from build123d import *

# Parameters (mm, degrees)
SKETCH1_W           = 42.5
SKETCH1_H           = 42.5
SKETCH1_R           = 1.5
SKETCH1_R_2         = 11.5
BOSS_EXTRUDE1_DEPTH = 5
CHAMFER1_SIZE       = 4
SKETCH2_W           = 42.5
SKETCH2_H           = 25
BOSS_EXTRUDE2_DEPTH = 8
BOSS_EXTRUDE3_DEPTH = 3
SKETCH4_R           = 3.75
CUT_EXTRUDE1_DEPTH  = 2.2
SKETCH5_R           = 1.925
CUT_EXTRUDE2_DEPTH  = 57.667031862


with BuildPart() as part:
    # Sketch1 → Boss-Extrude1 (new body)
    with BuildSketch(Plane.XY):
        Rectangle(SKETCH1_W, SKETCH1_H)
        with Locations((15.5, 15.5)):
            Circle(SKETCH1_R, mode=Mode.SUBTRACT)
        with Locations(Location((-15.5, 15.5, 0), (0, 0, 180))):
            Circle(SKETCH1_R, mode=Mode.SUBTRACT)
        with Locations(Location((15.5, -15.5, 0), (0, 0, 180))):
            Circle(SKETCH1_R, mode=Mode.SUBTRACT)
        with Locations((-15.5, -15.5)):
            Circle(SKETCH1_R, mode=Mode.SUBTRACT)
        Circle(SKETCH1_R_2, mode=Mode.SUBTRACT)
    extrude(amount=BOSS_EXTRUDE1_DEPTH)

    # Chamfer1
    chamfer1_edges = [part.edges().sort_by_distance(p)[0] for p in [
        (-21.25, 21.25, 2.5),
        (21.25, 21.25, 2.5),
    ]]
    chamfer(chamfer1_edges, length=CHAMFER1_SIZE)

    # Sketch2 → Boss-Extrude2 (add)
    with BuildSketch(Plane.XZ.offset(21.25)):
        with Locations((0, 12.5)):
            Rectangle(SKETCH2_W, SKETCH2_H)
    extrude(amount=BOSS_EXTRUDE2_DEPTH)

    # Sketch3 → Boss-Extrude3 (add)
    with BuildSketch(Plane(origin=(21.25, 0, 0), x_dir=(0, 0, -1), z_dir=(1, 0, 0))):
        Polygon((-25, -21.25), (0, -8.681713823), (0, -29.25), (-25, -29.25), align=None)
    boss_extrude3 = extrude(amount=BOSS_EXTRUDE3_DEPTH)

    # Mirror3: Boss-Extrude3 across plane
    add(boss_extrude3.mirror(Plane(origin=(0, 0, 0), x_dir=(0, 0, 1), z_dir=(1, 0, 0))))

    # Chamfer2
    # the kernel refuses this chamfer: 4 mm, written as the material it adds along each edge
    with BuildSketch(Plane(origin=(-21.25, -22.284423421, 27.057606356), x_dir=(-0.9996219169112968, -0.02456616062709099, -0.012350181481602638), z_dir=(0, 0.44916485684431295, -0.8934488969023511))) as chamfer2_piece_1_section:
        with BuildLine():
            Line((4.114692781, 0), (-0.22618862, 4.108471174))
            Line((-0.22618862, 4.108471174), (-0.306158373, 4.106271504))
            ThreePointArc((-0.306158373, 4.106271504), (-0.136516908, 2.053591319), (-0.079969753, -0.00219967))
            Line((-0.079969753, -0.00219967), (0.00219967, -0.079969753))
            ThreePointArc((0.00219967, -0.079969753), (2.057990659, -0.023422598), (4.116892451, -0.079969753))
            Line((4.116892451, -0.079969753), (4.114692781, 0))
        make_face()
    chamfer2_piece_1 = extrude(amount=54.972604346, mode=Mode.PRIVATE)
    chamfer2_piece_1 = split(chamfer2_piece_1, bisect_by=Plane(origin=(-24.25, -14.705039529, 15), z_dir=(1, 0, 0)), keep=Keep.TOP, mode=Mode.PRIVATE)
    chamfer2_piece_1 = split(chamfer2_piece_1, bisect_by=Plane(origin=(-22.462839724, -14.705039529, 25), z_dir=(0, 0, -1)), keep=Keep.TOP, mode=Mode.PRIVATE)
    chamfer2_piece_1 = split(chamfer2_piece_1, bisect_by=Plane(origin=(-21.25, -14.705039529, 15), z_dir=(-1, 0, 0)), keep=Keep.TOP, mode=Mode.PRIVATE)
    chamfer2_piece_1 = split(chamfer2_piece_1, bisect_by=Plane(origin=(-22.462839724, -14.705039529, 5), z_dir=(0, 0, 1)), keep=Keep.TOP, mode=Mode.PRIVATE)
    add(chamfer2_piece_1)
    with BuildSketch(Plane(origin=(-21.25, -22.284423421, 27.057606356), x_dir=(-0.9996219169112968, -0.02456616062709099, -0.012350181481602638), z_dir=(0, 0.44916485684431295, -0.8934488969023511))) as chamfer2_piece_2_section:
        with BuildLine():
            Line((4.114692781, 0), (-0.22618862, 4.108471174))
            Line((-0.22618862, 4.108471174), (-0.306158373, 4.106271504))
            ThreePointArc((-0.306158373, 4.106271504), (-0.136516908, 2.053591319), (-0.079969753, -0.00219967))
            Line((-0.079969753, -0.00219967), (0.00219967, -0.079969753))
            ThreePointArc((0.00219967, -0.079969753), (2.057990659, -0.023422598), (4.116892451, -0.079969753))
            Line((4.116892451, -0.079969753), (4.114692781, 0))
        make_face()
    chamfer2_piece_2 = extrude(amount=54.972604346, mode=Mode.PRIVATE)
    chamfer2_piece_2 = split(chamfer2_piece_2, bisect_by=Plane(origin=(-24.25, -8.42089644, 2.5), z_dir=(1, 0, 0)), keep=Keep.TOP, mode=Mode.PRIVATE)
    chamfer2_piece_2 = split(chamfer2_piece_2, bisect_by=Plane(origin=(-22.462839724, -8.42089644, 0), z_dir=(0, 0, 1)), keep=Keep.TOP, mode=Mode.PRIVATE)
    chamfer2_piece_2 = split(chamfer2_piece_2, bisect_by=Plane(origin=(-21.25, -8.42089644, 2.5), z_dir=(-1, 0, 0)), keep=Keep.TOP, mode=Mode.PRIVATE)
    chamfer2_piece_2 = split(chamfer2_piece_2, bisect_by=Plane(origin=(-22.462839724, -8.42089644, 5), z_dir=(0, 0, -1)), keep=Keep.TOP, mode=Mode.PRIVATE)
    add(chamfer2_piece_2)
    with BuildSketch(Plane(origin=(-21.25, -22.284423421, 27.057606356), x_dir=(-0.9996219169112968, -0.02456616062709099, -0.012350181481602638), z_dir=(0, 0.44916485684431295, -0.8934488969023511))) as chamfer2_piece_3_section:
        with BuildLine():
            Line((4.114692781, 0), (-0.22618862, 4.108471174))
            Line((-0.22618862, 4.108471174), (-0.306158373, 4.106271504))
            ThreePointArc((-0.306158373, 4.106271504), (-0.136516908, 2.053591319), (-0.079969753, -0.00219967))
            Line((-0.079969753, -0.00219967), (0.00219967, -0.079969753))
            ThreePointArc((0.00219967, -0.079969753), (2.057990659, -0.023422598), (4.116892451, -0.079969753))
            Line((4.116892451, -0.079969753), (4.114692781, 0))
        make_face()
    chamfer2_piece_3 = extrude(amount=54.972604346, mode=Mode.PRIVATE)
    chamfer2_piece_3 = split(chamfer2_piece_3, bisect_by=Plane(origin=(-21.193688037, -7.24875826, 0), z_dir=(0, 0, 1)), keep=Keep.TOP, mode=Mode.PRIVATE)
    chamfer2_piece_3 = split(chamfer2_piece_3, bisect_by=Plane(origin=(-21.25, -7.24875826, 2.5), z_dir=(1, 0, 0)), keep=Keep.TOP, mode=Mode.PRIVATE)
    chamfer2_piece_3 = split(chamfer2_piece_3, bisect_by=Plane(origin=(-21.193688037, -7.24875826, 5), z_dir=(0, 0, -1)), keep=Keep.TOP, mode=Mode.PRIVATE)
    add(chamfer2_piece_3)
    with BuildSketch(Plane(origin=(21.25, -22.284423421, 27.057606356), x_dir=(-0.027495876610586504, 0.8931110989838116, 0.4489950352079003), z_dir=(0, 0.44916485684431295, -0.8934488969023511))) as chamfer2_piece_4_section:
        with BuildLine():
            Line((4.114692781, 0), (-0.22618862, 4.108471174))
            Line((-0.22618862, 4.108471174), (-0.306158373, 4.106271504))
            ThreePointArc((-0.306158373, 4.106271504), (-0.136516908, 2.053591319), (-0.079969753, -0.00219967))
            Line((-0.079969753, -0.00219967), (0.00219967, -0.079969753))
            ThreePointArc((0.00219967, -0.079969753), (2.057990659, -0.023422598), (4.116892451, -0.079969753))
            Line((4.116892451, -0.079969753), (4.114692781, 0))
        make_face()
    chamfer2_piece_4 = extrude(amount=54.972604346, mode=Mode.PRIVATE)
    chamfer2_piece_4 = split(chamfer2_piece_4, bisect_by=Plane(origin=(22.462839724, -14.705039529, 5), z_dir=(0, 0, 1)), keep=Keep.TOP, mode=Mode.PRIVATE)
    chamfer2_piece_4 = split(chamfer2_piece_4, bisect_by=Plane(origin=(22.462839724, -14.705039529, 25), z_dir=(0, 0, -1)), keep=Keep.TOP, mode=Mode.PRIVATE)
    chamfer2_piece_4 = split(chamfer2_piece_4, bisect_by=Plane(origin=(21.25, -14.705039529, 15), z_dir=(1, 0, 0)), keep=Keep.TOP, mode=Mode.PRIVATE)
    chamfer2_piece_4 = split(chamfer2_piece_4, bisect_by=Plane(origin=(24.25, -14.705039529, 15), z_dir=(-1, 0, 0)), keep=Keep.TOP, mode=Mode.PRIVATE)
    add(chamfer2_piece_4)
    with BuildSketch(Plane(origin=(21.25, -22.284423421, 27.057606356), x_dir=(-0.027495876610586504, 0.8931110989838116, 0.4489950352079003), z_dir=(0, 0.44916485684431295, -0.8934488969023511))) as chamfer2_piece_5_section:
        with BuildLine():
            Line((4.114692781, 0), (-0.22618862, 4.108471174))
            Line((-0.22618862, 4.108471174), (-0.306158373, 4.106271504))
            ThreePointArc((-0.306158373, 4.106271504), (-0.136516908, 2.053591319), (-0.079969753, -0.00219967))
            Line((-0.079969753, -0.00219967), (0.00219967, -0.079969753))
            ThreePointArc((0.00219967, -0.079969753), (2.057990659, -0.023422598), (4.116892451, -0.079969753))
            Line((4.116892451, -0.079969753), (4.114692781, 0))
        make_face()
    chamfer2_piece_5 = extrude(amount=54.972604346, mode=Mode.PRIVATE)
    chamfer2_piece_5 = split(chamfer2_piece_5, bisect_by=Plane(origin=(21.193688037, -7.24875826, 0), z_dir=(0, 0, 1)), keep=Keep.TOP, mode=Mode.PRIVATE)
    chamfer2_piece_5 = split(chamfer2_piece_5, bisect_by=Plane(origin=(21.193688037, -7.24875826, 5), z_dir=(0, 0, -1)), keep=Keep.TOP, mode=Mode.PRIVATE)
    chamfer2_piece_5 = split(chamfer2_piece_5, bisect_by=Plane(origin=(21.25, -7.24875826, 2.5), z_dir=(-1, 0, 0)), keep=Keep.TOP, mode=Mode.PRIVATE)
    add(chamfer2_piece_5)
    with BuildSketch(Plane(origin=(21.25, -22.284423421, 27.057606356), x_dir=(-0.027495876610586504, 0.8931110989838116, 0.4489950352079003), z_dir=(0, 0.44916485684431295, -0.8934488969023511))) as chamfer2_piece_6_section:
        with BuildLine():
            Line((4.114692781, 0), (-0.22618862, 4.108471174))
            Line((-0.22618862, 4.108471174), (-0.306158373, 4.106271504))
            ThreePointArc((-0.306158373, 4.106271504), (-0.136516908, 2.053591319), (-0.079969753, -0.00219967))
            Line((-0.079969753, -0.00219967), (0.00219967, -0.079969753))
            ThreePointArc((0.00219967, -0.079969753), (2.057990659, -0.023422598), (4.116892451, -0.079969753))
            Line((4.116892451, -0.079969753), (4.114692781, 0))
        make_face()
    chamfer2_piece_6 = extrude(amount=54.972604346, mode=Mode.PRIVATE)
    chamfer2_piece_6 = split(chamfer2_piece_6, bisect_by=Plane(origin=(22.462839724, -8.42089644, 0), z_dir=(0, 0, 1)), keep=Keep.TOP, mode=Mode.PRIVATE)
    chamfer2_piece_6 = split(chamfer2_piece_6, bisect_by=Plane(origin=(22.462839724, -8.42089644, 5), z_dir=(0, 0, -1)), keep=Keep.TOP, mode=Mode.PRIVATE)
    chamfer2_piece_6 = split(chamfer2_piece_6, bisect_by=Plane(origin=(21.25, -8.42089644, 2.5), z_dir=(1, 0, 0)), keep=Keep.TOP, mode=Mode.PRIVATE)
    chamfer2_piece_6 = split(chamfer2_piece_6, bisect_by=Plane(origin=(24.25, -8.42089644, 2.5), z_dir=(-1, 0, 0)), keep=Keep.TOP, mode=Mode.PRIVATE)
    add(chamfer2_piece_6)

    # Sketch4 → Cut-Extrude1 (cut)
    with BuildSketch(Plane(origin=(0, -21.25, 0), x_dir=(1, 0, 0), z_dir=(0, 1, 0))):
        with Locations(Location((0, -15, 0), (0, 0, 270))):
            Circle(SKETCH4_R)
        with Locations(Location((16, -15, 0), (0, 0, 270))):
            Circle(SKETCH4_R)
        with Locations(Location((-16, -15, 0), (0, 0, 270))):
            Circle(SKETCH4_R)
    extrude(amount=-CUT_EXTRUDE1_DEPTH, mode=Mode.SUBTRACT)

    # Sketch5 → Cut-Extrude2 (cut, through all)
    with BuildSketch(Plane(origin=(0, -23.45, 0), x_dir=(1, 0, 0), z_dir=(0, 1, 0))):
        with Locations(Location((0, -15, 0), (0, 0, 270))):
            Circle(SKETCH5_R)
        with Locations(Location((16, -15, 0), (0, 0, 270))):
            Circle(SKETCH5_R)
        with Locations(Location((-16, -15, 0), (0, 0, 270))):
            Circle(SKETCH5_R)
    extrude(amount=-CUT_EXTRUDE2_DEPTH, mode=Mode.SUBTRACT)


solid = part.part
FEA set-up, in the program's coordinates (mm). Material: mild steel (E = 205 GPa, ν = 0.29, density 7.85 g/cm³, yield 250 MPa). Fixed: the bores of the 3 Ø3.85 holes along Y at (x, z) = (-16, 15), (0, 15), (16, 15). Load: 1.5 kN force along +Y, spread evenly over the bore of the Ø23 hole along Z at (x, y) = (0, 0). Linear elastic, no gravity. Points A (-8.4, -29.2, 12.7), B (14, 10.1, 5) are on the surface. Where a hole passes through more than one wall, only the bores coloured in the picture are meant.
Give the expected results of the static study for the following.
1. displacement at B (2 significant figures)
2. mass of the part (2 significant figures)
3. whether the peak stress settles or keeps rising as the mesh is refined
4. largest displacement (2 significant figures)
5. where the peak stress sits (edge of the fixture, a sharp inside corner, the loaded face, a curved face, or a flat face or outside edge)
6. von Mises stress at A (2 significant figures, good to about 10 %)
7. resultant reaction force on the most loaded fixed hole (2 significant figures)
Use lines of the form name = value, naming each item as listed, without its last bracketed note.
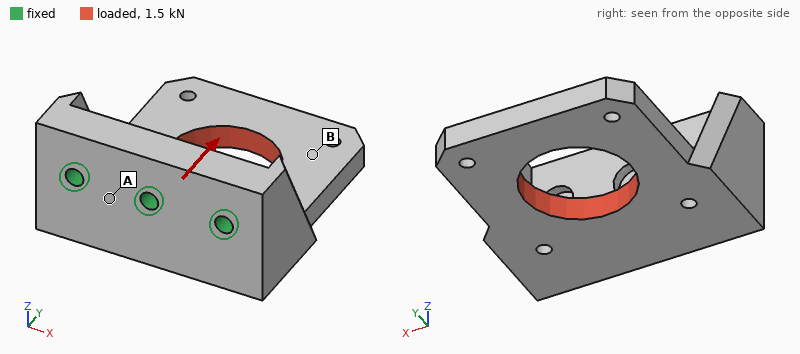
displacement at B = 15 µm
mass of the part = 140 g
whether the peak stress settles or keeps rising as the mesh is refined = keeps rising
largest displacement = 21 µm
where the peak stress sits = edge of the fixture
von Mises stress at A = 16 MPa
resultant reaction force on the most loaded fixed hole = 540 N
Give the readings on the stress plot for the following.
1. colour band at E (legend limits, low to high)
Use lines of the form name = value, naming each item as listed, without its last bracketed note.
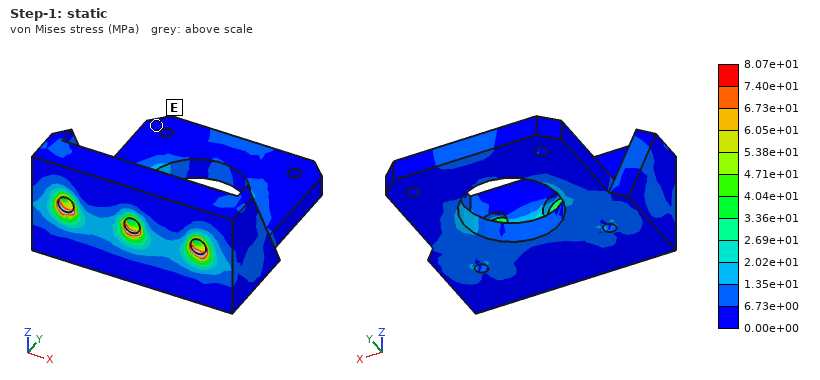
colour band at E = 0.00e+00 to 6.73e+00 MPa
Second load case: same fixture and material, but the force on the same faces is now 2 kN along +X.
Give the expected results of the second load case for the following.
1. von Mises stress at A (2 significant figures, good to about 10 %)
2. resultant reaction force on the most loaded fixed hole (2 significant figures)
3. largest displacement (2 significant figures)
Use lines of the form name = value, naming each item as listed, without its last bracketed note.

von Mises stress at A = 16 MPa
resultant reaction force on the most loaded fixed hole = 1.7 kN
largest displacement = 35 µm
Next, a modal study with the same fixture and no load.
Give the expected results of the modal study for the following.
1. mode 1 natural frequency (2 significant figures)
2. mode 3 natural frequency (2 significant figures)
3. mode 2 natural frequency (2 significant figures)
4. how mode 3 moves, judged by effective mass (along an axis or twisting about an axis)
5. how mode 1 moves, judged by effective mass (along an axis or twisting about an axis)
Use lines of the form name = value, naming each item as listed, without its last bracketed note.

mode 1 natural frequency = 2200 Hz
mode 3 natural frequency = 7100 Hz
mode 2 natural frequency = 4900 Hz
how mode 3 moves, judged by effective mass = along X
how mode 1 moves, judged by effective mass = along Z
